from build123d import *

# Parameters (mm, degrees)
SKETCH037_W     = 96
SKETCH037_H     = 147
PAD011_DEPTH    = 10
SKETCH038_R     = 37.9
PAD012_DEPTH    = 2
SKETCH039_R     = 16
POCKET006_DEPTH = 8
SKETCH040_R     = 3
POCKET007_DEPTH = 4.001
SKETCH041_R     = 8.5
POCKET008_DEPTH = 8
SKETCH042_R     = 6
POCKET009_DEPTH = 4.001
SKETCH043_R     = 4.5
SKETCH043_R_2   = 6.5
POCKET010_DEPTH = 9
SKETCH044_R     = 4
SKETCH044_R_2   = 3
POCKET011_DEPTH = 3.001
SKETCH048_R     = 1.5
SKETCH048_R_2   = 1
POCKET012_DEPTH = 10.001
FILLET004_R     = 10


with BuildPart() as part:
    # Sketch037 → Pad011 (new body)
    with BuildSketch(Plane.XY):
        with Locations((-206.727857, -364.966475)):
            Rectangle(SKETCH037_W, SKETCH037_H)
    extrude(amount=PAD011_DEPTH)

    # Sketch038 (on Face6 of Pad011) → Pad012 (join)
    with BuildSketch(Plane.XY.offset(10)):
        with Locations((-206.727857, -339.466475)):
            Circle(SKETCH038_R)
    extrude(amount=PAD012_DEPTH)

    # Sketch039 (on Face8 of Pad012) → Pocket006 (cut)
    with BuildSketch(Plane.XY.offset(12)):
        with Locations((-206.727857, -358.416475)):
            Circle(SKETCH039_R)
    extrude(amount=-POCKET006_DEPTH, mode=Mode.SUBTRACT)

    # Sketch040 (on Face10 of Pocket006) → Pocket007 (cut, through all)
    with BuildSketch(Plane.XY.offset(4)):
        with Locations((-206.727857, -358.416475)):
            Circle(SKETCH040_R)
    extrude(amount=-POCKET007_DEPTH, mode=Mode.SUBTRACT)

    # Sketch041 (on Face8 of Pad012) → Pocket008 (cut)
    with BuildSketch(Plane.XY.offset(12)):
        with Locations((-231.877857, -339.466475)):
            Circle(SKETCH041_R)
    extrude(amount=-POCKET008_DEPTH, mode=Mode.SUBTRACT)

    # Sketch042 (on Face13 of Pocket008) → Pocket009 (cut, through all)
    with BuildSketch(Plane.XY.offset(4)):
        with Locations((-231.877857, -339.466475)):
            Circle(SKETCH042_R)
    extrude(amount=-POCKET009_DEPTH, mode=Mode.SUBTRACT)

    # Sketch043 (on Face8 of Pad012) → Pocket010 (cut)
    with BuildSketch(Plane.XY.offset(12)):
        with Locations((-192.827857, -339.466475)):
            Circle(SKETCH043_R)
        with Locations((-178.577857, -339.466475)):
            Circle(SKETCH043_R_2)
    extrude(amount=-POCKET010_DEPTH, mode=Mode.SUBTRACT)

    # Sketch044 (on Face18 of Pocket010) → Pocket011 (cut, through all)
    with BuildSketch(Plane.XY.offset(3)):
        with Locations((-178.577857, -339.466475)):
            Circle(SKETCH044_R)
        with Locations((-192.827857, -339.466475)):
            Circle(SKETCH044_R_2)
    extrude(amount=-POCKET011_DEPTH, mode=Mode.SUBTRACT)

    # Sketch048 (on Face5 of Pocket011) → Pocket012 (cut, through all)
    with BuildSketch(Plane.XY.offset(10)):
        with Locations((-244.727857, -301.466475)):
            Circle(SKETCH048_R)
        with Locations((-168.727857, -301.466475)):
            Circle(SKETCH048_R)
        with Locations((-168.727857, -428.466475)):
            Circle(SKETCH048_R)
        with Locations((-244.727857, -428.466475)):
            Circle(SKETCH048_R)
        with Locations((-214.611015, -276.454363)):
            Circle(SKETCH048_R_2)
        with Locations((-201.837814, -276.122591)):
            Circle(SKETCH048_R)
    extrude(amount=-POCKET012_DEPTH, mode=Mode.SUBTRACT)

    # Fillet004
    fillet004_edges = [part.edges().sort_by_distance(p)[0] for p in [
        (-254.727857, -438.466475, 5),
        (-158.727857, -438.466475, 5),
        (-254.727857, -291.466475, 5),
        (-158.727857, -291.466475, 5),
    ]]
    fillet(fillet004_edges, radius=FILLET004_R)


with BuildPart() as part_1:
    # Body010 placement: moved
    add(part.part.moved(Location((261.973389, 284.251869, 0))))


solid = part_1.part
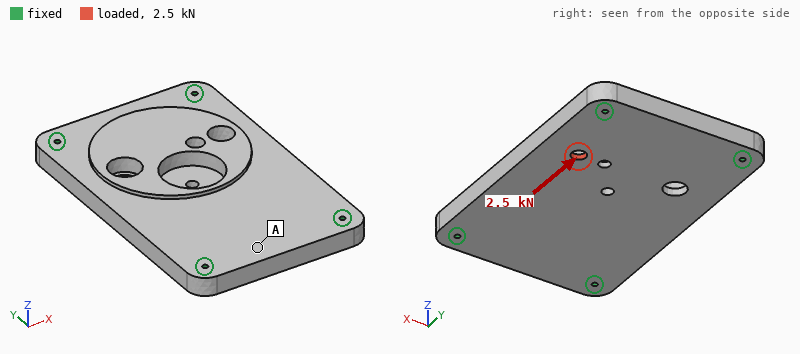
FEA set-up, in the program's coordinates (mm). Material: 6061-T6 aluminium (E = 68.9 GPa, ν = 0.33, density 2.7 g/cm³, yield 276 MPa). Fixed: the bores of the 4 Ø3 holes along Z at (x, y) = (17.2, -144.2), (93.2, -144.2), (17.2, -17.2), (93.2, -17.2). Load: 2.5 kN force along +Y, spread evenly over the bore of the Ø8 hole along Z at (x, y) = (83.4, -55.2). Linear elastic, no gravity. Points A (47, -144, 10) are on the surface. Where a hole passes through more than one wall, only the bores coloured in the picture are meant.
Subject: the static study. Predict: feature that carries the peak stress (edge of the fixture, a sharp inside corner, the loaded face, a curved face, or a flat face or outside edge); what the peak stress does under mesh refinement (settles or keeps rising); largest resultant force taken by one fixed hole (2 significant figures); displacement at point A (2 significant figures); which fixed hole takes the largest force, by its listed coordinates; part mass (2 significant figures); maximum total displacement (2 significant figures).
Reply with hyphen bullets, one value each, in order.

- a sharp inside corner
- keeps rising
- 1.2 kN
- 1.4 µm
- (93.2, -17.2)
- 370 g
- 9.0 µm
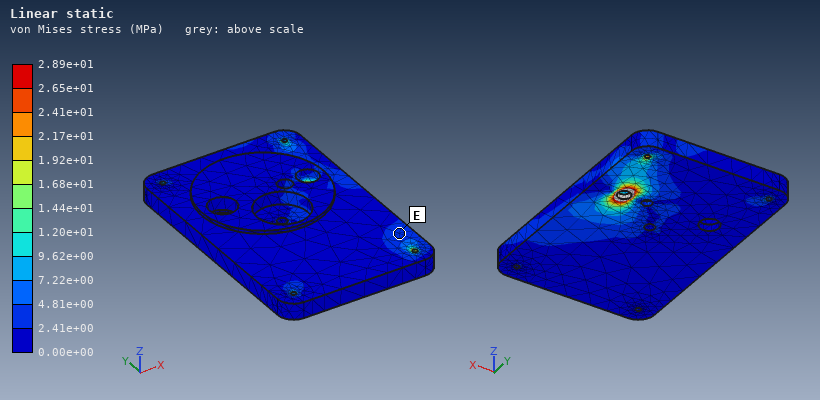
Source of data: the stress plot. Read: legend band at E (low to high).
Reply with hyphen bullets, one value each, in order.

- 2.41e+00 to 4.81e+00 MPa
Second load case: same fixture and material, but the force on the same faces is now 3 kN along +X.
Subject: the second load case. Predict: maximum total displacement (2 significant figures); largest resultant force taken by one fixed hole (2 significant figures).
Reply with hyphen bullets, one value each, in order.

- 15 µm
- 1.2 kN
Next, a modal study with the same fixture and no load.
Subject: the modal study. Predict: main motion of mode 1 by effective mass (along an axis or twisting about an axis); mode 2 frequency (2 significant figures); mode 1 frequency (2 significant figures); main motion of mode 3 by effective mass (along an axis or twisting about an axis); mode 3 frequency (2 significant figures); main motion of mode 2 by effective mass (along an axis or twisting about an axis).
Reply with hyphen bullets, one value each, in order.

- along Z
- 3800 Hz
- 2400 Hz
- twisting about X
- 5800 Hz
- twisting about Y
